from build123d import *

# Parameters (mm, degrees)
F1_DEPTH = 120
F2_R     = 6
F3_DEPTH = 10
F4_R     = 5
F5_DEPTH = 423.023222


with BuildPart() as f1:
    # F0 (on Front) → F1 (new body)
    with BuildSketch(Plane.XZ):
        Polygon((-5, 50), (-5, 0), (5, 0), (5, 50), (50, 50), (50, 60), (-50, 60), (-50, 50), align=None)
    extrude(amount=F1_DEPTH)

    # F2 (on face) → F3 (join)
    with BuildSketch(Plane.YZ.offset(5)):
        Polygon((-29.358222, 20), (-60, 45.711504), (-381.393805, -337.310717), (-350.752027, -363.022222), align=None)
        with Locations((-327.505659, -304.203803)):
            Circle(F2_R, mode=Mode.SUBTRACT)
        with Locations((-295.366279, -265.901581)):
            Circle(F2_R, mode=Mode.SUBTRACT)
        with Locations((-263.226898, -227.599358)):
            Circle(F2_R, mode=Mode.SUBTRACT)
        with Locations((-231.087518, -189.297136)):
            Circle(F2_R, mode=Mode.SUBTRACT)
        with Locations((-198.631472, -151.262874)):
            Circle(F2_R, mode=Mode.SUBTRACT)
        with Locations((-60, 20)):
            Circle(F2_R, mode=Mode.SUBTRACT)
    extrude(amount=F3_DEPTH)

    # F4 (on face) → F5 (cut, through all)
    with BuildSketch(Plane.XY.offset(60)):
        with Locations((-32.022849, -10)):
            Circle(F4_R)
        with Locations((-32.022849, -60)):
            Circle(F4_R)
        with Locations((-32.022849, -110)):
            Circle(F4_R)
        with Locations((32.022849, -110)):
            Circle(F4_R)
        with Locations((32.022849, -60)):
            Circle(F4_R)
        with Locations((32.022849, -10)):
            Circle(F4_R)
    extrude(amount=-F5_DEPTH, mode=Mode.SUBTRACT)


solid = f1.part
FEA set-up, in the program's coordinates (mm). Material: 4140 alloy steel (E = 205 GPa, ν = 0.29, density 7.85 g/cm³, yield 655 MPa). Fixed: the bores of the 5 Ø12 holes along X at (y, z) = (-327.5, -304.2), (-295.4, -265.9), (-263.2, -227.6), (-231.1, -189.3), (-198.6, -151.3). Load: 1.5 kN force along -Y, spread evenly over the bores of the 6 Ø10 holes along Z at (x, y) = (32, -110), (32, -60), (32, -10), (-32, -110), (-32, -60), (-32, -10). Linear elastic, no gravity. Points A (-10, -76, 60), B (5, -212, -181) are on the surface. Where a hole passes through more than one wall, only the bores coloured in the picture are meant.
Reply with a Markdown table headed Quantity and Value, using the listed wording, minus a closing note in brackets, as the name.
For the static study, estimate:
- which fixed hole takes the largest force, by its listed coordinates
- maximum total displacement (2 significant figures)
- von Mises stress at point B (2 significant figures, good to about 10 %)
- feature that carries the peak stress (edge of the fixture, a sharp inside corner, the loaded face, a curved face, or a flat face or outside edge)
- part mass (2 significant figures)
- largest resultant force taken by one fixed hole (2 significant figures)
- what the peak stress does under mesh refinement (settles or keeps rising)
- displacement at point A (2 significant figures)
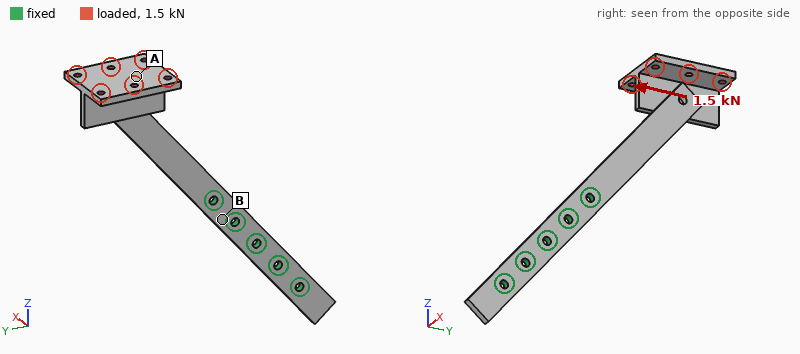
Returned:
| Quantity | Value |
|---|---|
| which fixed hole takes the largest force, by its listed coordinates | (-198.6, -151.3) |
| maximum total displacement | 1.1 mm |
| von Mises stress at point B | 20 MPa |
| feature that carries the peak stress | edge of the fixture |
| part mass | 2.9 kg |
| largest resultant force taken by one fixed hole | 4.4 kN |
| what the peak stress does under mesh refinement | keeps rising |
| displacement at point A | 0.79 mm |
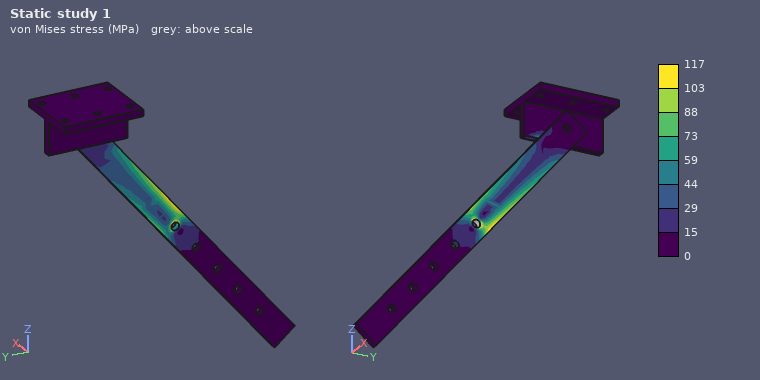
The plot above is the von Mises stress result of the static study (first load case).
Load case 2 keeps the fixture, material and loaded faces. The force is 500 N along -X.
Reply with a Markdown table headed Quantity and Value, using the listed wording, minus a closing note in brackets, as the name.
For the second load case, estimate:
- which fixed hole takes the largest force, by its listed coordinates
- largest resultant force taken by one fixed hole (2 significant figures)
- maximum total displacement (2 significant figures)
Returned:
| Quantity | Value |
|---|---|
| which fixed hole takes the largest force, by its listed coordinates | (-198.6, -151.3) |
| largest resultant force taken by one fixed hole | 740 N |
| maximum total displacement | 4.5 mm |
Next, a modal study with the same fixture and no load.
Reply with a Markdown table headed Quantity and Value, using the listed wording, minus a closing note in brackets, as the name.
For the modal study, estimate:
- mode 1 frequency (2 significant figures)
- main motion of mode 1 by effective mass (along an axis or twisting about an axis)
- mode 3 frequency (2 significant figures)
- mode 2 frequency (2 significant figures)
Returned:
| Quantity | Value |
|---|---|
| mode 1 frequency | 49 Hz |
| main motion of mode 1 by effective mass | along X |
| mode 3 frequency | 240 Hz |
| mode 2 frequency | 170 Hz |
